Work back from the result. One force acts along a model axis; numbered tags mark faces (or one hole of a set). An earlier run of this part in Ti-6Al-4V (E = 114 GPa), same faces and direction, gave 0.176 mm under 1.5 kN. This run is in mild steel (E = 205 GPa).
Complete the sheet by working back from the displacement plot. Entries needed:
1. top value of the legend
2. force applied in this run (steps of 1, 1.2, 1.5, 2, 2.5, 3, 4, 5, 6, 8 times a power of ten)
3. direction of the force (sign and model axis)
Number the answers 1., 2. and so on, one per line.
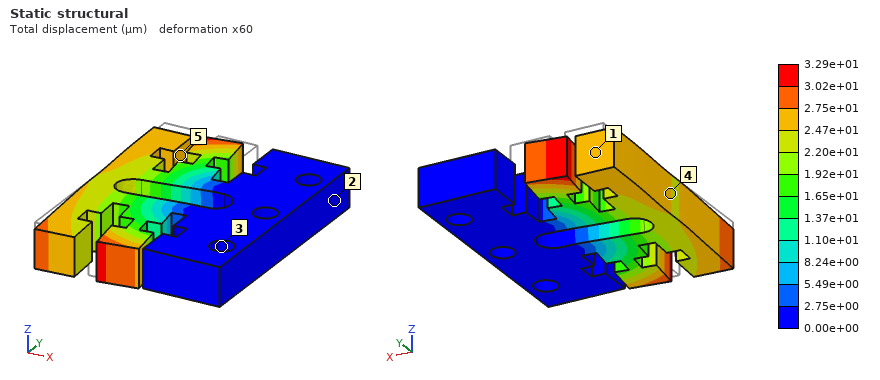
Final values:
1. 3.29e+01 µm
2. 500 N
3. -Y
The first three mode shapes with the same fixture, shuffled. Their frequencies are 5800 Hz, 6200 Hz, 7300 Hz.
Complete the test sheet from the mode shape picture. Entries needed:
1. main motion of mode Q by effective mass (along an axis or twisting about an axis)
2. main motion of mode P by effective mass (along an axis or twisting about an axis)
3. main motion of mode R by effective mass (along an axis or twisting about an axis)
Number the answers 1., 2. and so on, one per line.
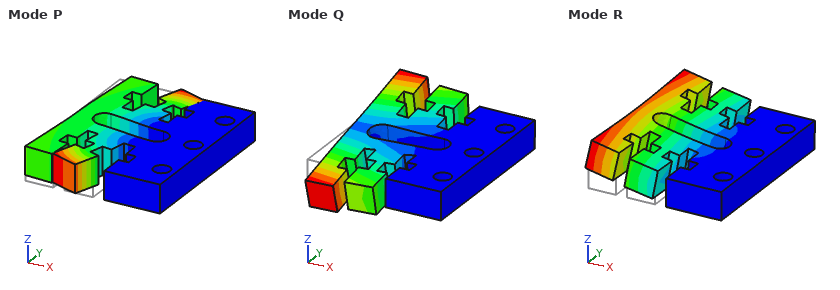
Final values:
1. twisting about X
2. along Y
3. along Z
